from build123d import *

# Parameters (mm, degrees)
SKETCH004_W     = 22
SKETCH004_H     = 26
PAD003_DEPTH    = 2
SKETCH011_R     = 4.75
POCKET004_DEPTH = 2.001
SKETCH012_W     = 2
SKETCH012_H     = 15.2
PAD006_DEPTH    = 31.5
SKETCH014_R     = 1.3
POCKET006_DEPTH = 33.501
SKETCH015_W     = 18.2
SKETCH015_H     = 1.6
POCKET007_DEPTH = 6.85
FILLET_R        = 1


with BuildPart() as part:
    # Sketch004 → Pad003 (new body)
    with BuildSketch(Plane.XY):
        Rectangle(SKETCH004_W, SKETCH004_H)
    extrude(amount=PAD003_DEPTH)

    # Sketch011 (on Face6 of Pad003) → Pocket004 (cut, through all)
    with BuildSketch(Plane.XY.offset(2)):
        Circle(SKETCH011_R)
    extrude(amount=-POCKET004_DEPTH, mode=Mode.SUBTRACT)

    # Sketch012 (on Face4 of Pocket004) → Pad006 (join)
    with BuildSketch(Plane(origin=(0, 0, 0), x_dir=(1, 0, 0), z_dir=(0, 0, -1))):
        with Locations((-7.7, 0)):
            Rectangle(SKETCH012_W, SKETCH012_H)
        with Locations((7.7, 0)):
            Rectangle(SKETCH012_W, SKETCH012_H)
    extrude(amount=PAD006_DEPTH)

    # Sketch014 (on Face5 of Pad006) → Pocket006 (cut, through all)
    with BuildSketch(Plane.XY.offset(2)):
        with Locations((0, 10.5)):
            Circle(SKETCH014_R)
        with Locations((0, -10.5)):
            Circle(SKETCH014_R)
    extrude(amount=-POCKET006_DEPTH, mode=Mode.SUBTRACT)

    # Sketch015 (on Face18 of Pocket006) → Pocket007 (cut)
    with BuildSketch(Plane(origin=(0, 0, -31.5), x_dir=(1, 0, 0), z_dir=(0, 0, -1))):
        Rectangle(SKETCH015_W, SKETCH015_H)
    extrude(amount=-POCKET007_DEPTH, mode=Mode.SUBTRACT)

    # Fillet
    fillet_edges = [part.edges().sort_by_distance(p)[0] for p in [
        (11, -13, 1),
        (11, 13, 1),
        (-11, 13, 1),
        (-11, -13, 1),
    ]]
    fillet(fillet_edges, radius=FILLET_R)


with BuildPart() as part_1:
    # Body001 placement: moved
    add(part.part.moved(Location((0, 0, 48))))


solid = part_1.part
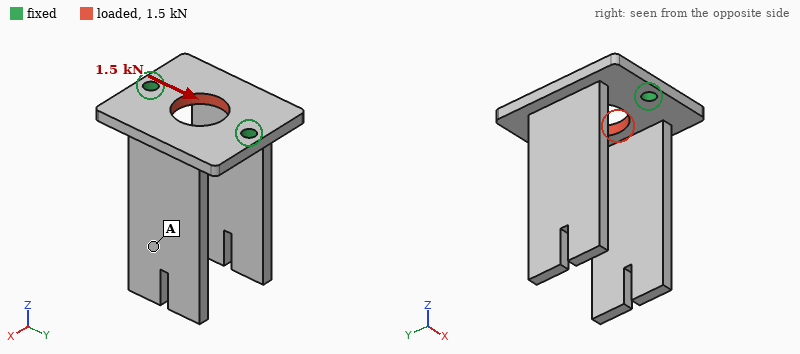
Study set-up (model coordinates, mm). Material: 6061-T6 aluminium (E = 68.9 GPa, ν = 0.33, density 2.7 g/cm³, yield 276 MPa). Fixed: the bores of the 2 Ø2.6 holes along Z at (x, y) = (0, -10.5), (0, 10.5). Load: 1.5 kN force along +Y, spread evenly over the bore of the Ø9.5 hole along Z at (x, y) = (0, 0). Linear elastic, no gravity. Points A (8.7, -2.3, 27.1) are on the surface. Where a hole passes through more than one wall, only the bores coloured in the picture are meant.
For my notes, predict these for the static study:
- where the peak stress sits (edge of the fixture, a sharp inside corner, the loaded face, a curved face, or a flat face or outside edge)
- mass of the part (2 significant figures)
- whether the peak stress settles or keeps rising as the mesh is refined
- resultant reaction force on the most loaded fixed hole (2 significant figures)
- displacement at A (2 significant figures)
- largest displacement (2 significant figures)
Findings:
edge of the fixture
7.7 g
keeps rising
750 N
3.9 µm
7.0 µm
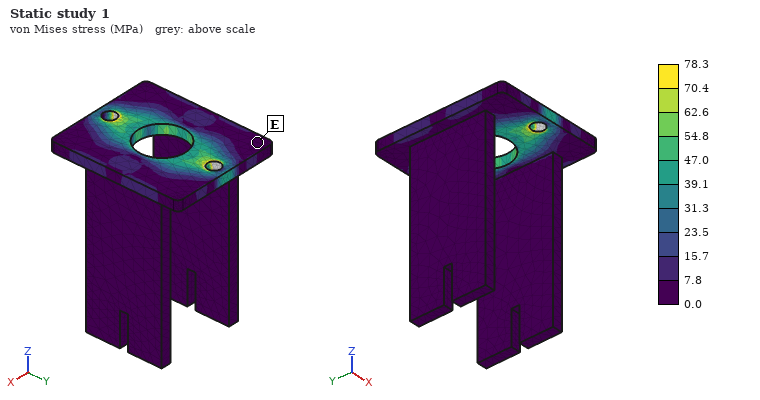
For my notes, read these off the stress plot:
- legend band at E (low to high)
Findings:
0.0 to 7.8 MPa
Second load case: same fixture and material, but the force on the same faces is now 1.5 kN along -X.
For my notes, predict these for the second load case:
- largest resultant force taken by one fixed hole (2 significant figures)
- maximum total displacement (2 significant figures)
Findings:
750 N
12 µm
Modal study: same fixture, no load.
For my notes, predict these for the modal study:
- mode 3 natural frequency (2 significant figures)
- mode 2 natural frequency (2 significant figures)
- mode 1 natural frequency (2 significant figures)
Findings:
4000 Hz
1200 Hz
1200 Hz
